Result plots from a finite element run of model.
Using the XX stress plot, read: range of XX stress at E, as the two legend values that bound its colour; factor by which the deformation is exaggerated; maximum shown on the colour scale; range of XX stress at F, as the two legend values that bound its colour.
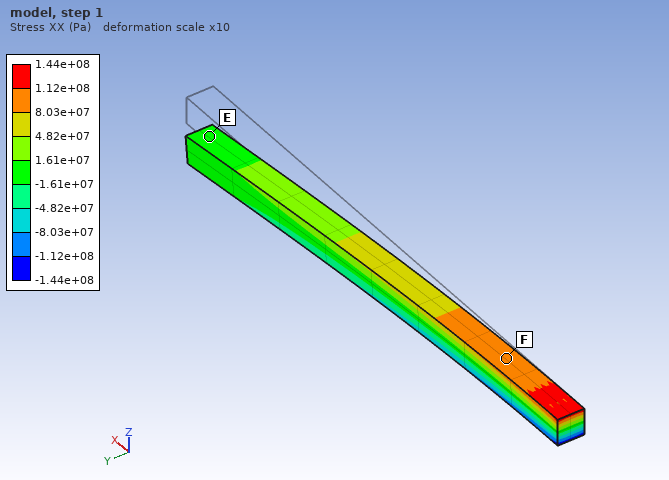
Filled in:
-1.61e+07 to 1.61e+07 Pa
10
1.44e+08 Pa
8.03e+07 to 1.12e+08 Pa
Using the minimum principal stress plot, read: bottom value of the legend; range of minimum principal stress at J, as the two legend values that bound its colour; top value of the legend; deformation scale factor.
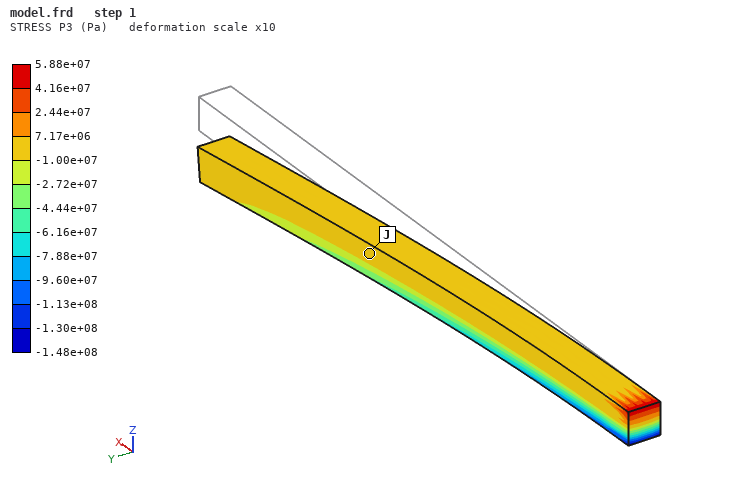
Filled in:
-1.48e+08 Pa
-1.00e+07 to 7.17e+06 Pa
5.88e+07 Pa
10
